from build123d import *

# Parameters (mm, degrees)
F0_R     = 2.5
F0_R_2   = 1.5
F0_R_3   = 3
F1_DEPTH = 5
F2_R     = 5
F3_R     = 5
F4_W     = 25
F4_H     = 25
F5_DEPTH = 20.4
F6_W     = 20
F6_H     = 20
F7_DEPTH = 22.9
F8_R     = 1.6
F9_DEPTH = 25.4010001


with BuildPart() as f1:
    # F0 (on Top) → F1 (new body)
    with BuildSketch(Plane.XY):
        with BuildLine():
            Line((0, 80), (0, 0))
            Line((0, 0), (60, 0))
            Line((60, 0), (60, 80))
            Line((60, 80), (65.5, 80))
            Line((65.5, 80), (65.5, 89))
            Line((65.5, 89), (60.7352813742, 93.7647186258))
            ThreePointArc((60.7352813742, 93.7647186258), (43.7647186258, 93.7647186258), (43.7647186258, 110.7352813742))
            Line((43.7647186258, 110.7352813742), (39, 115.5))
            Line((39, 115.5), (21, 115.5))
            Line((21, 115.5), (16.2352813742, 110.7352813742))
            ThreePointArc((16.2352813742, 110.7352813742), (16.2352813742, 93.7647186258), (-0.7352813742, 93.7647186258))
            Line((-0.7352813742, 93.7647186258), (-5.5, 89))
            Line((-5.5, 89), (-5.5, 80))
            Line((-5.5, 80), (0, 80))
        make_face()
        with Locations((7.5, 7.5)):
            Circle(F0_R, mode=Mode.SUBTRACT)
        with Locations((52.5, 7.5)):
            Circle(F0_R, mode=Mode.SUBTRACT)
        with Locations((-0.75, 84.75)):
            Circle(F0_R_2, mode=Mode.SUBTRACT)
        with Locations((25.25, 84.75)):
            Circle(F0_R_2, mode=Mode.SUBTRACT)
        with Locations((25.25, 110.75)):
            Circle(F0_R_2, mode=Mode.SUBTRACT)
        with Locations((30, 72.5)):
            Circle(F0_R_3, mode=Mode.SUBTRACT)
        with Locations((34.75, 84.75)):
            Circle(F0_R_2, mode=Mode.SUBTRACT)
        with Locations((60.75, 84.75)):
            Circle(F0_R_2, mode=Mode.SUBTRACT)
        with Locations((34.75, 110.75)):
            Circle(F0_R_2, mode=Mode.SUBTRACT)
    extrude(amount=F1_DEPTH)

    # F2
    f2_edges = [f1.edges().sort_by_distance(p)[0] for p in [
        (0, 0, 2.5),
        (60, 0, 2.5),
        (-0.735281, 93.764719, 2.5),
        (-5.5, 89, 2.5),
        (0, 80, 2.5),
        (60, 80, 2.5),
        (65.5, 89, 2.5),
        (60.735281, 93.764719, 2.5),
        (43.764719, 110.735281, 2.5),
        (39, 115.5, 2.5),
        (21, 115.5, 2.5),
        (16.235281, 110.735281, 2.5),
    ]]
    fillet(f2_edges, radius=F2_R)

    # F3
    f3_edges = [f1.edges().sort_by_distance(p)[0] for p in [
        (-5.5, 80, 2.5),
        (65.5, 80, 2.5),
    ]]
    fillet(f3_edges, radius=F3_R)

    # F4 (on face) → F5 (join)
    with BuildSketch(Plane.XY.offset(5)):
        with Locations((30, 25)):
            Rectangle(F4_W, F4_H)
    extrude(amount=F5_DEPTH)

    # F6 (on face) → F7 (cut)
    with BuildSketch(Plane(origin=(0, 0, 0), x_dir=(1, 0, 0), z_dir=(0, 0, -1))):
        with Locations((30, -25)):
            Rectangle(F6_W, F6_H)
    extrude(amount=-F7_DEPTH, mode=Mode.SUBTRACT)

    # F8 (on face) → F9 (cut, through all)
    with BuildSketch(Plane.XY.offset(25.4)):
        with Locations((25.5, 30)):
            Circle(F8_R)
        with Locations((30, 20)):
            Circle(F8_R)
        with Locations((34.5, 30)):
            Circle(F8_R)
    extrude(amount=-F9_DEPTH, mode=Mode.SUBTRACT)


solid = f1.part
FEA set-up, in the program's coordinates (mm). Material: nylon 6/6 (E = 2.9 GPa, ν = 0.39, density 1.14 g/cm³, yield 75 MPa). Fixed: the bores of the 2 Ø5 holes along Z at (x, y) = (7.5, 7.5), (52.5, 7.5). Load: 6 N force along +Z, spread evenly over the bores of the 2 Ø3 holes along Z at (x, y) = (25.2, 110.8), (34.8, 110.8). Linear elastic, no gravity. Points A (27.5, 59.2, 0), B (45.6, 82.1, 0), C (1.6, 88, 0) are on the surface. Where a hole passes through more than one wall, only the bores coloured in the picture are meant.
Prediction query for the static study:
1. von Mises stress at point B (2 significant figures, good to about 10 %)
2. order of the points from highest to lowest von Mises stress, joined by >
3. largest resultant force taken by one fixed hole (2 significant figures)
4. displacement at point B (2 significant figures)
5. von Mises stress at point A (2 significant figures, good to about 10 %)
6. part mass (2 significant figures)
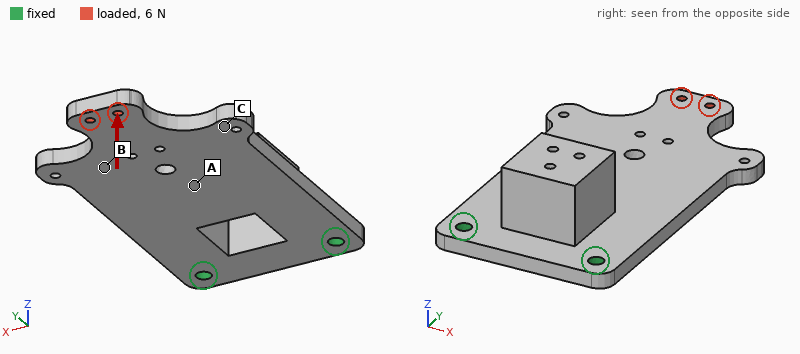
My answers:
0.89 MPa
A > B > C
3.1 N
0.66 mm
1.1 MPa
38 g
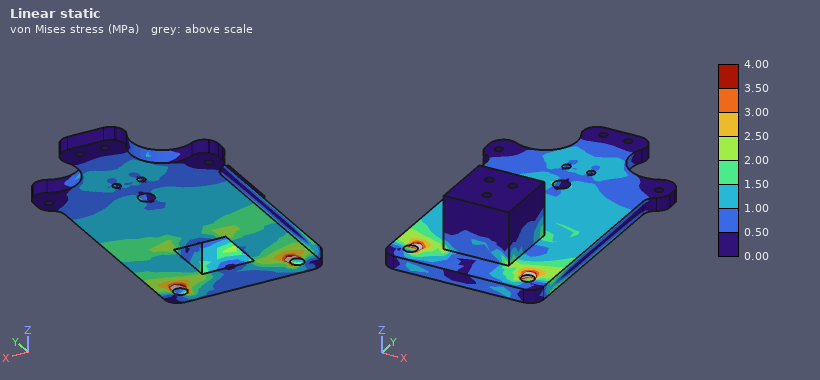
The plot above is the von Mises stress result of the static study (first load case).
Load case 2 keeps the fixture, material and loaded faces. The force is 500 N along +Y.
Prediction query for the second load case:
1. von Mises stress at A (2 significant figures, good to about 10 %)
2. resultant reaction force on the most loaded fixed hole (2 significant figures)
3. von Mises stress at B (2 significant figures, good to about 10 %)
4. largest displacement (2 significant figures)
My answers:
1.6 MPa
250 N
2.3 MPa
0.16 mm
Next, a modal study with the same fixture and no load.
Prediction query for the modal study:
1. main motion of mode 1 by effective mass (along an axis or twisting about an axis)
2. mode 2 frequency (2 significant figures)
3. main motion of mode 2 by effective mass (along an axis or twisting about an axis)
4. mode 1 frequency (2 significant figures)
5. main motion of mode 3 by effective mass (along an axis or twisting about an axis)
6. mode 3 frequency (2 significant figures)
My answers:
along Z
610 Hz
twisting about Y
150 Hz
along Z
710 Hz
